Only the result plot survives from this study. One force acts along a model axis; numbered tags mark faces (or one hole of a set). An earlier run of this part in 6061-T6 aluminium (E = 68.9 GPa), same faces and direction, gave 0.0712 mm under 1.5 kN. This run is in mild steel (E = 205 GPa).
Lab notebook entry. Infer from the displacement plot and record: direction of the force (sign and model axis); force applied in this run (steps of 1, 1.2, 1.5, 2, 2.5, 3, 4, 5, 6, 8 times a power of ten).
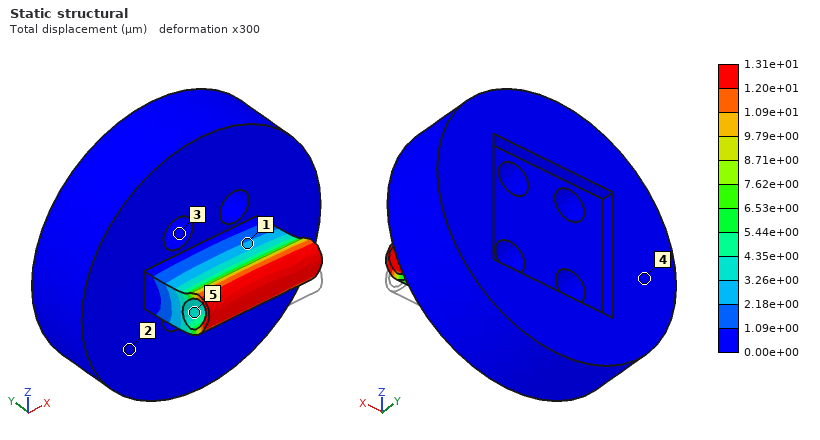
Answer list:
+Z
800 N
